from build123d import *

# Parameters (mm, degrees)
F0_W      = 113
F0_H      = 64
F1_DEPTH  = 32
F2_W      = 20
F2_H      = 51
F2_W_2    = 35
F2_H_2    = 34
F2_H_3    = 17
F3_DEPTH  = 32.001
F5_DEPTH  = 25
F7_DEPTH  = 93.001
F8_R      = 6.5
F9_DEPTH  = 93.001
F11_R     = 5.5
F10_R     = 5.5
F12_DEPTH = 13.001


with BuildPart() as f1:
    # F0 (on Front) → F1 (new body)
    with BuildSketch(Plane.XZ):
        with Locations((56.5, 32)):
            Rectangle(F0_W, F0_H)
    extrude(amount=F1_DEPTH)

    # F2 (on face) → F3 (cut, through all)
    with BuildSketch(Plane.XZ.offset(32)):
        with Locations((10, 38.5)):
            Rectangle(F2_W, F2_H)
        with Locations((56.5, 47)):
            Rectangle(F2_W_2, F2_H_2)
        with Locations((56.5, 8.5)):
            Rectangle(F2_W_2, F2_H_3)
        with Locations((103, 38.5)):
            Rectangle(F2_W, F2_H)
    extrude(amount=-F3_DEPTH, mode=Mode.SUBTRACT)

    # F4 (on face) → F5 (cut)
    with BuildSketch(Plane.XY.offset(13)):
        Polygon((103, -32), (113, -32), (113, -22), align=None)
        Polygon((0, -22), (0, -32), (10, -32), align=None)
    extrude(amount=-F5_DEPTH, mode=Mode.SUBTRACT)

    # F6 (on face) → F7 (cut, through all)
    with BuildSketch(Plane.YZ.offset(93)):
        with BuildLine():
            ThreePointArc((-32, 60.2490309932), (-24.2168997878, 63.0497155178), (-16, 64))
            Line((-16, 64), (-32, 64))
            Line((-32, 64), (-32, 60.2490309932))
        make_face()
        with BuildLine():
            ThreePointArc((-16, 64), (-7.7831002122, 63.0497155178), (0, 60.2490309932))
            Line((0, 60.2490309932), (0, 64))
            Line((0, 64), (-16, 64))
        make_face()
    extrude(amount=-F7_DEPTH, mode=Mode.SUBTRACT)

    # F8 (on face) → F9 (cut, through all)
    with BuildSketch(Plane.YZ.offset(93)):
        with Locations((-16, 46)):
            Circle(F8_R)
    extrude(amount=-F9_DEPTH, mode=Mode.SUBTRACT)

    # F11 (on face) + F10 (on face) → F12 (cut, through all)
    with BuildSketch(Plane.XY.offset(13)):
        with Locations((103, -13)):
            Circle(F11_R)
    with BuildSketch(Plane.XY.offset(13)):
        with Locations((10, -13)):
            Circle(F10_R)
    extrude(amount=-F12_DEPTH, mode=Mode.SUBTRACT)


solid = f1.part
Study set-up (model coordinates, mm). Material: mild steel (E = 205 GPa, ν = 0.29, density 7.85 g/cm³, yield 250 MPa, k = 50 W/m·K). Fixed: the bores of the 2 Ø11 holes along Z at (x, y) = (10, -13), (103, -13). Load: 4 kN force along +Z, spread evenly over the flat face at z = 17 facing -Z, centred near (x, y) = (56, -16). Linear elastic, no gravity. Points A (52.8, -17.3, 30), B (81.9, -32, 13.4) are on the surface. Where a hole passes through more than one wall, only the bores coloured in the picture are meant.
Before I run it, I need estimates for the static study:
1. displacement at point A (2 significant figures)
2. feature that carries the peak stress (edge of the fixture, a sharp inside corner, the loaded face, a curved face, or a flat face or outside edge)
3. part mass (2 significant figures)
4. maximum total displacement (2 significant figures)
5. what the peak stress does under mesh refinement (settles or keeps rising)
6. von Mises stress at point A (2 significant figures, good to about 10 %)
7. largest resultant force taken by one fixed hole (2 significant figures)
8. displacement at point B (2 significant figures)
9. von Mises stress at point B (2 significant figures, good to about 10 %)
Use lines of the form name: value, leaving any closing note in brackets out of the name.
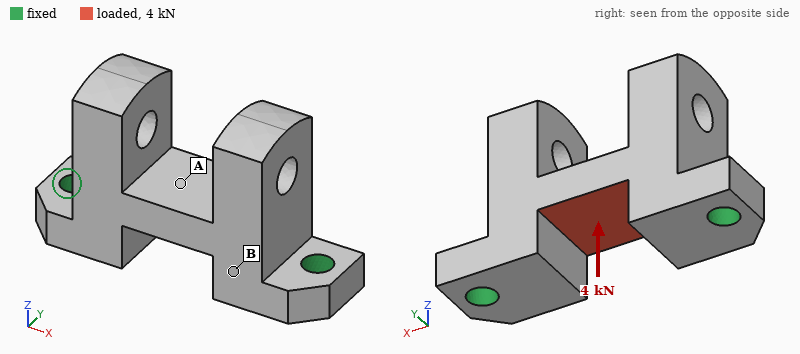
displacement at point A: 5.0 µm
feature that carries the peak stress: edge of the fixture
part mass: 770 g
maximum total displacement: 6.3 µm
what the peak stress does under mesh refinement: keeps rising
von Mises stress at point A: 19 MPa
largest resultant force taken by one fixed hole: 3.1 kN
displacement at point B: 2.9 µm
von Mises stress at point B: 7.0 MPa
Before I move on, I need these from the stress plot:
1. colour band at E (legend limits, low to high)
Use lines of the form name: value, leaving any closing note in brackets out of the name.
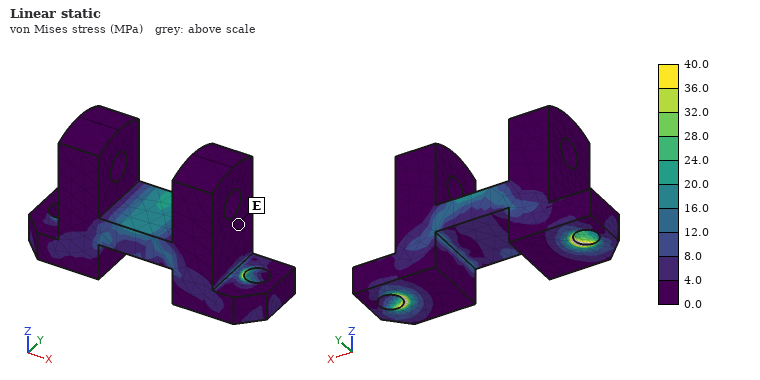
colour band at E: 0.0 to 4.0 MPa
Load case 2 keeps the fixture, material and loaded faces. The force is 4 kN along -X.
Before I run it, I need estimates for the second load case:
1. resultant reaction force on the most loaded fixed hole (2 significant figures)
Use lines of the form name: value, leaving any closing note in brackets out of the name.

resultant reaction force on the most loaded fixed hole: 2.0 kN
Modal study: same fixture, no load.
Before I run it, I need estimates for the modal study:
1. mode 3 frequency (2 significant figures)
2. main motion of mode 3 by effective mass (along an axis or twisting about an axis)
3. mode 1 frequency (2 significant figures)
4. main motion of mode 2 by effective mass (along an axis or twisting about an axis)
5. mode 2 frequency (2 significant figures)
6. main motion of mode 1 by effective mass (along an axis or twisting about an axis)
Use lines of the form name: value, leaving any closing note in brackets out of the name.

mode 3 frequency: 5500 Hz
main motion of mode 3 by effective mass: along X
mode 1 frequency: 3000 Hz
main motion of mode 2 by effective mass: twisting about Z
mode 2 frequency: 4500 Hz
main motion of mode 1 by effective mass: along Y
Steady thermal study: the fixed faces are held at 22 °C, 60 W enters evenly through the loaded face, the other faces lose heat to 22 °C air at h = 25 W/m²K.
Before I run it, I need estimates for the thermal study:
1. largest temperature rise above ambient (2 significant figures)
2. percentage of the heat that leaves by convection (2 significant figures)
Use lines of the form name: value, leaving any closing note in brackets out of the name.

largest temperature rise above ambient: 49 K
percentage of the heat that leaves by convection: 18 %
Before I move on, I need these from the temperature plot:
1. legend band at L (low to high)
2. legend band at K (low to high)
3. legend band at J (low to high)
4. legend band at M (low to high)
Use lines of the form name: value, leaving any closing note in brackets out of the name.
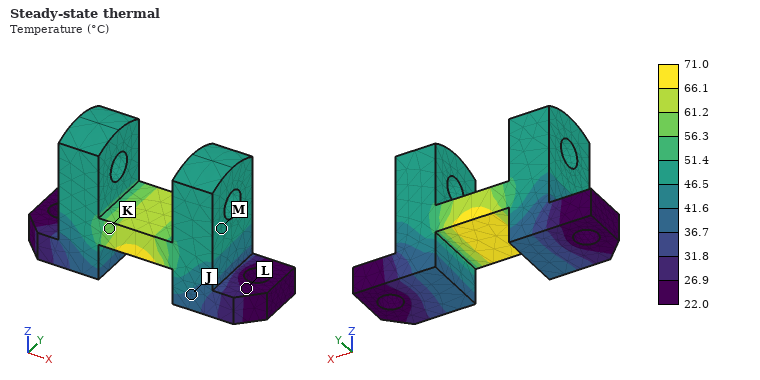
legend band at L: 22.0 to 26.9 °C
legend band at K: 56.3 to 61.2 °C
legend band at J: 36.7 to 41.6 °C
legend band at M: 46.5 to 51.4 °C
